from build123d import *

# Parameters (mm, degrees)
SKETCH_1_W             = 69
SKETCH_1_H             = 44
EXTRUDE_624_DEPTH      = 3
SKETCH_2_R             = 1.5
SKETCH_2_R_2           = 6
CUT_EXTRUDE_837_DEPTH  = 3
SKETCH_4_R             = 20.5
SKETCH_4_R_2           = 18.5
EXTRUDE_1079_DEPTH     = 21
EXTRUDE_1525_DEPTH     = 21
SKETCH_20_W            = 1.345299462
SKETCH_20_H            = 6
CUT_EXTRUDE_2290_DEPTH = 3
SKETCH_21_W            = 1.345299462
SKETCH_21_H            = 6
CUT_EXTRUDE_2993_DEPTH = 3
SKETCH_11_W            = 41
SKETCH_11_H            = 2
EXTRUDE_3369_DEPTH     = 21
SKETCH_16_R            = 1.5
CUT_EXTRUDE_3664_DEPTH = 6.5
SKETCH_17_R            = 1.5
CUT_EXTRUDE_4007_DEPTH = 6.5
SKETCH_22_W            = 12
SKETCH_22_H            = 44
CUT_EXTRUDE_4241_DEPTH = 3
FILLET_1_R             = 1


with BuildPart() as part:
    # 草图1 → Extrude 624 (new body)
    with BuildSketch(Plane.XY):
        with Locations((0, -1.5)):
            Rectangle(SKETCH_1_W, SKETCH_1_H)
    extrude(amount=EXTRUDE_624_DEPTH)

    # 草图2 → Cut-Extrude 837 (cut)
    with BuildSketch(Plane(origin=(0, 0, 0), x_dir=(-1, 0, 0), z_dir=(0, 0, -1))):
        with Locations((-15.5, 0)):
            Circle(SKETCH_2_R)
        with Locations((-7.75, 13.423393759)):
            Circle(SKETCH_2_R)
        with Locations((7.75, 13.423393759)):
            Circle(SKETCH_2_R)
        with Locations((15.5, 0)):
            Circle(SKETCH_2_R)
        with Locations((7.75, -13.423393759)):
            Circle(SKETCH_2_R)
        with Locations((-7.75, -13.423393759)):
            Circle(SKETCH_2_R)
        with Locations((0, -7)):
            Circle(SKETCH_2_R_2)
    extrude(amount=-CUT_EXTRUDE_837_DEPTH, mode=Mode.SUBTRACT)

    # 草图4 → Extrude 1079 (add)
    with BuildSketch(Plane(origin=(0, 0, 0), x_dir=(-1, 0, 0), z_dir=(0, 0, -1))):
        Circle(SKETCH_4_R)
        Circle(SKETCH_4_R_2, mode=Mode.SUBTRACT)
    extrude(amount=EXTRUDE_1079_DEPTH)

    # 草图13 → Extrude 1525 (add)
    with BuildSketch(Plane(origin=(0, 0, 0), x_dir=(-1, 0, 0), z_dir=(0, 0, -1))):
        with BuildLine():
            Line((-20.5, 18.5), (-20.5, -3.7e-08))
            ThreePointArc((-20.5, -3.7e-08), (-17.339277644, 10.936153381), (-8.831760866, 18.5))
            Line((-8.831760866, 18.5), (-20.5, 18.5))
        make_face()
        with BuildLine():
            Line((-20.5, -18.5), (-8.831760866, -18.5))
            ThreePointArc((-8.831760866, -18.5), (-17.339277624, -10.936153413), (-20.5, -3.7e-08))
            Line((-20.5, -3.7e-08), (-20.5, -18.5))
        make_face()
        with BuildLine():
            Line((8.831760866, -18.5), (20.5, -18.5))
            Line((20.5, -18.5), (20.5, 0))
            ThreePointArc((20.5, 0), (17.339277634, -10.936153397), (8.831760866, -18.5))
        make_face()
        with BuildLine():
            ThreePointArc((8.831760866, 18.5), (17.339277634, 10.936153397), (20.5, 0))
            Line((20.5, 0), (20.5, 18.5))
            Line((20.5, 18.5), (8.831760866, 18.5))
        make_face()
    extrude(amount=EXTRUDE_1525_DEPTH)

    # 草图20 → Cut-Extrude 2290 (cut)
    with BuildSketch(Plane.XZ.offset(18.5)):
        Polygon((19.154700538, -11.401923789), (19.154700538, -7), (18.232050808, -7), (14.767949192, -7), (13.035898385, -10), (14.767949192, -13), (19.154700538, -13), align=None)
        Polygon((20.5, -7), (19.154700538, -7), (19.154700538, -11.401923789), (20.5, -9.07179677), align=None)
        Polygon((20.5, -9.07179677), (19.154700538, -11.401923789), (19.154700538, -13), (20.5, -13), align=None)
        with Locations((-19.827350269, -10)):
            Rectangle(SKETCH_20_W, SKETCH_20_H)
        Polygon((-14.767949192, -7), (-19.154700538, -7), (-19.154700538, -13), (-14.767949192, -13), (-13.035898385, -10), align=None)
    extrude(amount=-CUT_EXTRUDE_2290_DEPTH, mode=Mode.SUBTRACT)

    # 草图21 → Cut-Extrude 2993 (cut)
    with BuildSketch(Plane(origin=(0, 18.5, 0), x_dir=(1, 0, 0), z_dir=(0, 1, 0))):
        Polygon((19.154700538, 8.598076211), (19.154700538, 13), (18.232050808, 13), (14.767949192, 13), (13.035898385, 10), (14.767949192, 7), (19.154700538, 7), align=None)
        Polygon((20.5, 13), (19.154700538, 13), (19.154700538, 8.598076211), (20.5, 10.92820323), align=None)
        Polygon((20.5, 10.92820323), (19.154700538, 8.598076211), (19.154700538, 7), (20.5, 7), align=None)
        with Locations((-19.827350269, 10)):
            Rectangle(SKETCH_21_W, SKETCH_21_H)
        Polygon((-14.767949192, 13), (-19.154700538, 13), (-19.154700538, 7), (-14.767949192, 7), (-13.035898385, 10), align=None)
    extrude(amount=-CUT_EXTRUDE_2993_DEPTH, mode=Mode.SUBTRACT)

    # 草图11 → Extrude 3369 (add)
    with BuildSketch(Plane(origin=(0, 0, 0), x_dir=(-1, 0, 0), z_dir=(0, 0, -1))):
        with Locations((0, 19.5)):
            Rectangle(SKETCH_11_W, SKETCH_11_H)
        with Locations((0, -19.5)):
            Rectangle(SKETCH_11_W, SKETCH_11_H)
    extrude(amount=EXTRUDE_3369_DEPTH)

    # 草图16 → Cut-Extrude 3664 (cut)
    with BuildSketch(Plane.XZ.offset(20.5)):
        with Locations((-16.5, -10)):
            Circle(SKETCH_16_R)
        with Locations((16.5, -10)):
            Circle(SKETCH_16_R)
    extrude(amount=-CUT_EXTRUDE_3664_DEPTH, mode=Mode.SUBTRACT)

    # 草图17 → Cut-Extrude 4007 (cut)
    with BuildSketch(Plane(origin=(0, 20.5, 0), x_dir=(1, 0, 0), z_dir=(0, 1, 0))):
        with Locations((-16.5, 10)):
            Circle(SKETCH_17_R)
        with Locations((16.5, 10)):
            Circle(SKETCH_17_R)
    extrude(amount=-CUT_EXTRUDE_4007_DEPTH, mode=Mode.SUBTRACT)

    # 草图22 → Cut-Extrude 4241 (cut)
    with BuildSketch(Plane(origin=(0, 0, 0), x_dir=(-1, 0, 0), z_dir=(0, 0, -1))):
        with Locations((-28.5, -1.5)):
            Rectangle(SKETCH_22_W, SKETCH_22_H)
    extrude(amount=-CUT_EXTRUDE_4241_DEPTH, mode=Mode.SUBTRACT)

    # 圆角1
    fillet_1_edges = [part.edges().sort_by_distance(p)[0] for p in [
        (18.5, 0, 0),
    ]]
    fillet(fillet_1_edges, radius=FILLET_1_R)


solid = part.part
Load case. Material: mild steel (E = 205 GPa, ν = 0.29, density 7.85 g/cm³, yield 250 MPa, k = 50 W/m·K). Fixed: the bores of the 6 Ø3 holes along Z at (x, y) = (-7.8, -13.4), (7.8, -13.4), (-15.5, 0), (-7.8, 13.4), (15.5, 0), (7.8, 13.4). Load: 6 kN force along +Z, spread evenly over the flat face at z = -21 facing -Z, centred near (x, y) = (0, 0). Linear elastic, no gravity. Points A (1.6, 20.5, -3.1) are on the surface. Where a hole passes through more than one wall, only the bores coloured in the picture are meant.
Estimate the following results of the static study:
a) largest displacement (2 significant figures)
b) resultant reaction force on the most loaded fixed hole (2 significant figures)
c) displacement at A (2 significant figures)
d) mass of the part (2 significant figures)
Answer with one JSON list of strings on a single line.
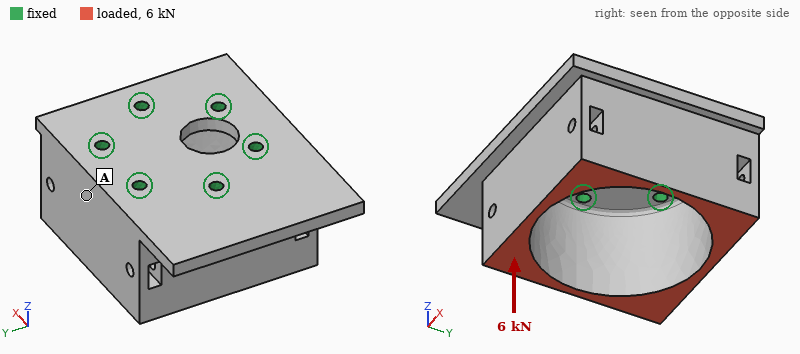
["7.2 µm", "1.1 kN", "3.6 µm", "150 g"]
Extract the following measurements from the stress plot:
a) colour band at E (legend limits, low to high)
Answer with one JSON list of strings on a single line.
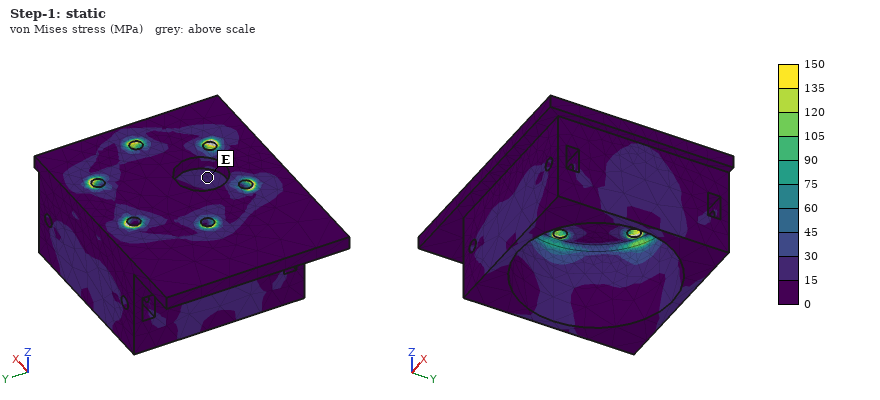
["15 to 30 MPa"]
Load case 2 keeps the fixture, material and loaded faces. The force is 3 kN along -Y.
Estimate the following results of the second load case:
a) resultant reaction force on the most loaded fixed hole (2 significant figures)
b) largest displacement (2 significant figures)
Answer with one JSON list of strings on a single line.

["1.2 kN", "16 µm"]
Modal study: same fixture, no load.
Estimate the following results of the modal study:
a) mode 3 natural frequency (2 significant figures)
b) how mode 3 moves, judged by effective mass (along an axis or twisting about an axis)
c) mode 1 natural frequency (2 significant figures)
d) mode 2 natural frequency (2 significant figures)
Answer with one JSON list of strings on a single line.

["9900 Hz", "along Y", "6800 Hz", "7600 Hz"]
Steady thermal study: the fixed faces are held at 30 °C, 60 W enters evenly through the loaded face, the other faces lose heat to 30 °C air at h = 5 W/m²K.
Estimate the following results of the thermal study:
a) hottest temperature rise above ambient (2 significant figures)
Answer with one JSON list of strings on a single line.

["68 K"]
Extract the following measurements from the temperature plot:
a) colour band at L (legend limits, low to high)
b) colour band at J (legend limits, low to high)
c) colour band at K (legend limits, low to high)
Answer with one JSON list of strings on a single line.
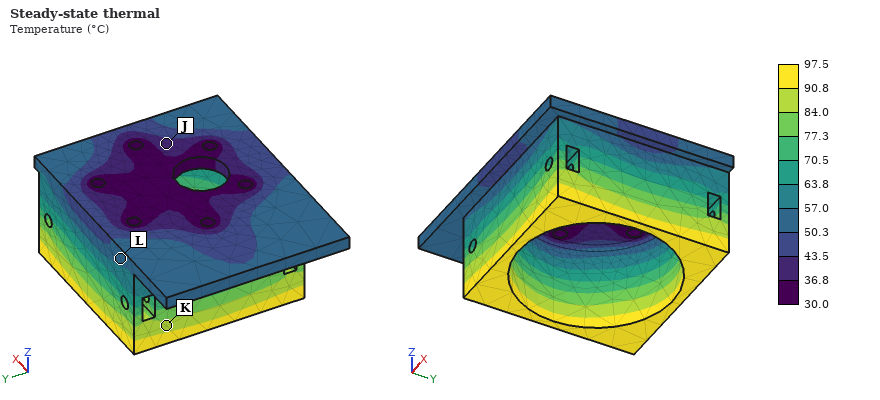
["50.3 to 57.0 °C", "36.8 to 43.5 °C", "84.0 to 90.8 °C"]
